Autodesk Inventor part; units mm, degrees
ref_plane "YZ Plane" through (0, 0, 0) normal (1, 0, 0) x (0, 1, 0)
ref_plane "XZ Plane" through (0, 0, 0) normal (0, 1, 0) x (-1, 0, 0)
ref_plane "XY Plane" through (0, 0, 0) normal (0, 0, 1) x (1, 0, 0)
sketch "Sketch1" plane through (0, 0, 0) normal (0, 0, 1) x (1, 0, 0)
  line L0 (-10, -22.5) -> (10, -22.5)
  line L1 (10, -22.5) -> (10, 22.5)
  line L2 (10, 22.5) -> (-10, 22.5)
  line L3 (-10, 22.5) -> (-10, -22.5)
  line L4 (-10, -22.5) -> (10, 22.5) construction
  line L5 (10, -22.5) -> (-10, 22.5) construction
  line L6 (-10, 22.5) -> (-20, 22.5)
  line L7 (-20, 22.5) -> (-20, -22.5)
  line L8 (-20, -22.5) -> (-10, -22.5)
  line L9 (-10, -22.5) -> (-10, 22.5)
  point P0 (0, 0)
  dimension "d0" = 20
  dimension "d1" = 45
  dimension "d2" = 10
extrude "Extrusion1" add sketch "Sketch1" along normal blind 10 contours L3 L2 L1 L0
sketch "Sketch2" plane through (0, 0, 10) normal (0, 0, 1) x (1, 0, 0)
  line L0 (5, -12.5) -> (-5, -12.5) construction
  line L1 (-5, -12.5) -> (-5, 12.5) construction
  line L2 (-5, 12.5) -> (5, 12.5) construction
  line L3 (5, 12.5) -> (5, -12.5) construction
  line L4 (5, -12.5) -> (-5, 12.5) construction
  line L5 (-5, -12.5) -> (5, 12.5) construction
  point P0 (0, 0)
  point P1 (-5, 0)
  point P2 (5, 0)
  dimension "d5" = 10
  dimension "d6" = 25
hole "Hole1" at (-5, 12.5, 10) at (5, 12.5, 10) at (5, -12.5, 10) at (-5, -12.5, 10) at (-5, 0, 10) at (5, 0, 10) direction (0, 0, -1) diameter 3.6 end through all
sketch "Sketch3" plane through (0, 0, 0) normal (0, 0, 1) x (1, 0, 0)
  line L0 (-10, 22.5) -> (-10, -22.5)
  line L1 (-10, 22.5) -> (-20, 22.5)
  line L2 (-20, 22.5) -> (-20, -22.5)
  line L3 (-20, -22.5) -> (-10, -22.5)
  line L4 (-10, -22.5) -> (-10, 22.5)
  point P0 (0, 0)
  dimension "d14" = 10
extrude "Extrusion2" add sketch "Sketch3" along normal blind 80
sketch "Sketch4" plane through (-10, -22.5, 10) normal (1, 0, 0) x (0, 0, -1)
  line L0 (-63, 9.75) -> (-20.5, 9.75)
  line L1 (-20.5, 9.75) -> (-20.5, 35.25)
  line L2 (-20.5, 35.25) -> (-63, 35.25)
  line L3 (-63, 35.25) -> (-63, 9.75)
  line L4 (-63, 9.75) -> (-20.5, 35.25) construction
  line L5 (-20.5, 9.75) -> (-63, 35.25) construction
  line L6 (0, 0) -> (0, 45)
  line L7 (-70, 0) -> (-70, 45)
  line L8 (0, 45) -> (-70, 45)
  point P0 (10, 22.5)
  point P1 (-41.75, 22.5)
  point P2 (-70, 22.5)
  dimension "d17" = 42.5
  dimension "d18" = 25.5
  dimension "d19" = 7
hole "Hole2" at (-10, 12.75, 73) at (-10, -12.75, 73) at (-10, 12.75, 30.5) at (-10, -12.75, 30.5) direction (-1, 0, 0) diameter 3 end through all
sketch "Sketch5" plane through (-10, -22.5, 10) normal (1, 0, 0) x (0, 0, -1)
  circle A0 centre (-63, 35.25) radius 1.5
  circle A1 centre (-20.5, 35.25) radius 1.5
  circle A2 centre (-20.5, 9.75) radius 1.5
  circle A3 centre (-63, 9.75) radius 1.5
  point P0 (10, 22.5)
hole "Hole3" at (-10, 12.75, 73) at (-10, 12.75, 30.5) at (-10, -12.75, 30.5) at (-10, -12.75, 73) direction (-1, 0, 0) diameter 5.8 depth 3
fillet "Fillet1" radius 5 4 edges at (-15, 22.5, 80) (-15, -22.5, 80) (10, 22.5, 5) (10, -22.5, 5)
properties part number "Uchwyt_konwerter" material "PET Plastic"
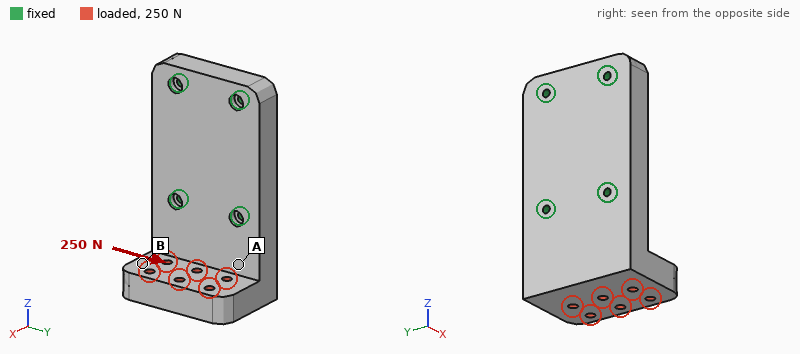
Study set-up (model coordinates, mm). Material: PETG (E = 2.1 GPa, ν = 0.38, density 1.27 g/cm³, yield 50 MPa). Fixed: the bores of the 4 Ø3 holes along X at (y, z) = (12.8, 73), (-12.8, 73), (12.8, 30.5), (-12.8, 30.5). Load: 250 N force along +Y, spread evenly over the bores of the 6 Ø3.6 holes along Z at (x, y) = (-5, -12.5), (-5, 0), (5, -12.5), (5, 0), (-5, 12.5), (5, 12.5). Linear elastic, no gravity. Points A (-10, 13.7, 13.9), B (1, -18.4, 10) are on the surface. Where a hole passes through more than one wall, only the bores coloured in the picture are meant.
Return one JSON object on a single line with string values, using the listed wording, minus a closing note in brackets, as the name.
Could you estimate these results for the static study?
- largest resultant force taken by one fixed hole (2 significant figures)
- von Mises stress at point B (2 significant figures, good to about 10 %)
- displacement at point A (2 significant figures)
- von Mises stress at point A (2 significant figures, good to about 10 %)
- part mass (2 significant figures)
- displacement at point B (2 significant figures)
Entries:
{"largest resultant force taken by one fixed hole": "270 N", "von Mises stress at point B": "0.86 MPa", "displacement at point A": "0.071 mm", "von Mises stress at point A": "3.8 MPa", "part mass": "55 g", "displacement at point B": "0.17 mm"}
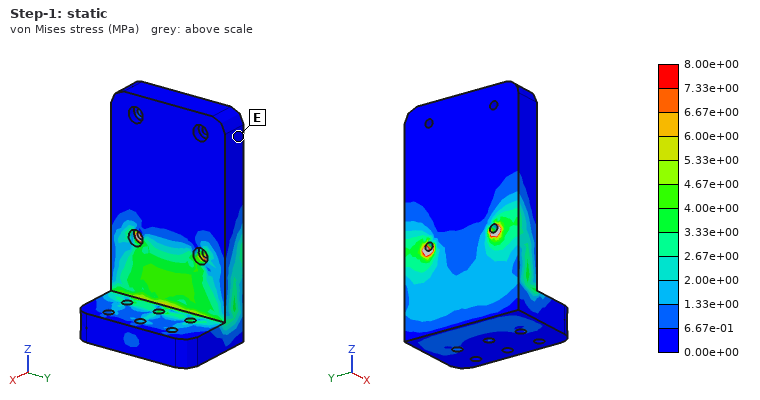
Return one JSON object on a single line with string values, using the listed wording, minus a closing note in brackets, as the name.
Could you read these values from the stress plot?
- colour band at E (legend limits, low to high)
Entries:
{"colour band at E": "0.00e+00 to 6.67e-01 MPa"}
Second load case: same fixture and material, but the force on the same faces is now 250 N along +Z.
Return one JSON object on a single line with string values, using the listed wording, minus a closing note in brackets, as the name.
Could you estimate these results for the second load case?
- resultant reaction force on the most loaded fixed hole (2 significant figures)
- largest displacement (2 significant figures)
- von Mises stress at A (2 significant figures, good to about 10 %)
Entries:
{"resultant reaction force on the most loaded fixed hole": "70 N", "largest displacement": "0.54 mm", "von Mises stress at A": "5.0 MPa"}
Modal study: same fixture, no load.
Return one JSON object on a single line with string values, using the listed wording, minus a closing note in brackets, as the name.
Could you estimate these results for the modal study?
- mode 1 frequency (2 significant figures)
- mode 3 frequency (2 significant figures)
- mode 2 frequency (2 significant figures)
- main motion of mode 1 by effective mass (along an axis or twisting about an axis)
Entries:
{"mode 1 frequency": "880 Hz", "mode 3 frequency": "2800 Hz", "mode 2 frequency": "1600 Hz", "main motion of mode 1 by effective mass": "along X"}
